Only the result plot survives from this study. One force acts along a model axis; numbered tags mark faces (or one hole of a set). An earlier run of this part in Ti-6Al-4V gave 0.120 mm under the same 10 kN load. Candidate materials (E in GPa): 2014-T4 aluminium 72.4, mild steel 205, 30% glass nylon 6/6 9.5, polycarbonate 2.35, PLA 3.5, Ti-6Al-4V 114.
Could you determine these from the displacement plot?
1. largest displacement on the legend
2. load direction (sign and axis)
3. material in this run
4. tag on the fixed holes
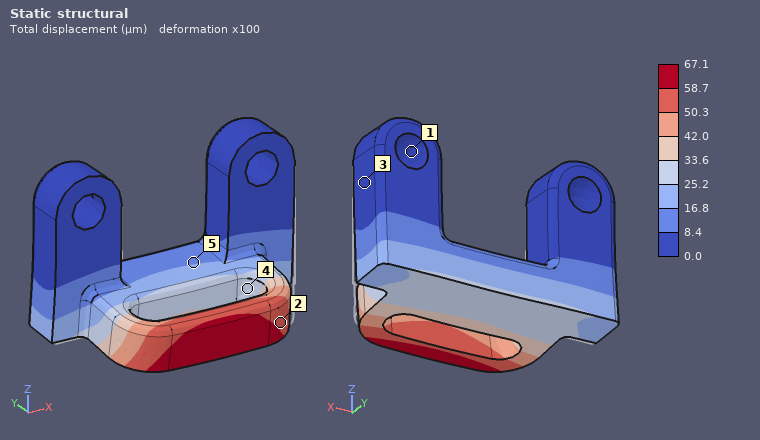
67.1 µm
-Z
mild steel
1
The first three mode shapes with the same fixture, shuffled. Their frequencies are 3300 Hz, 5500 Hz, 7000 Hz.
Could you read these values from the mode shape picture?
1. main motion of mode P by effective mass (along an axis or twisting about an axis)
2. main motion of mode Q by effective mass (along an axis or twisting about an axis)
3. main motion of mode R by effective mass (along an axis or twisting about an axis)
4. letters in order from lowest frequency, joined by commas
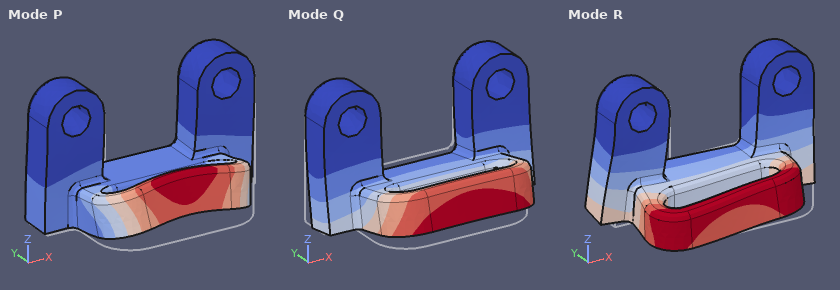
along Y
along Y
along X
Q, R, P
